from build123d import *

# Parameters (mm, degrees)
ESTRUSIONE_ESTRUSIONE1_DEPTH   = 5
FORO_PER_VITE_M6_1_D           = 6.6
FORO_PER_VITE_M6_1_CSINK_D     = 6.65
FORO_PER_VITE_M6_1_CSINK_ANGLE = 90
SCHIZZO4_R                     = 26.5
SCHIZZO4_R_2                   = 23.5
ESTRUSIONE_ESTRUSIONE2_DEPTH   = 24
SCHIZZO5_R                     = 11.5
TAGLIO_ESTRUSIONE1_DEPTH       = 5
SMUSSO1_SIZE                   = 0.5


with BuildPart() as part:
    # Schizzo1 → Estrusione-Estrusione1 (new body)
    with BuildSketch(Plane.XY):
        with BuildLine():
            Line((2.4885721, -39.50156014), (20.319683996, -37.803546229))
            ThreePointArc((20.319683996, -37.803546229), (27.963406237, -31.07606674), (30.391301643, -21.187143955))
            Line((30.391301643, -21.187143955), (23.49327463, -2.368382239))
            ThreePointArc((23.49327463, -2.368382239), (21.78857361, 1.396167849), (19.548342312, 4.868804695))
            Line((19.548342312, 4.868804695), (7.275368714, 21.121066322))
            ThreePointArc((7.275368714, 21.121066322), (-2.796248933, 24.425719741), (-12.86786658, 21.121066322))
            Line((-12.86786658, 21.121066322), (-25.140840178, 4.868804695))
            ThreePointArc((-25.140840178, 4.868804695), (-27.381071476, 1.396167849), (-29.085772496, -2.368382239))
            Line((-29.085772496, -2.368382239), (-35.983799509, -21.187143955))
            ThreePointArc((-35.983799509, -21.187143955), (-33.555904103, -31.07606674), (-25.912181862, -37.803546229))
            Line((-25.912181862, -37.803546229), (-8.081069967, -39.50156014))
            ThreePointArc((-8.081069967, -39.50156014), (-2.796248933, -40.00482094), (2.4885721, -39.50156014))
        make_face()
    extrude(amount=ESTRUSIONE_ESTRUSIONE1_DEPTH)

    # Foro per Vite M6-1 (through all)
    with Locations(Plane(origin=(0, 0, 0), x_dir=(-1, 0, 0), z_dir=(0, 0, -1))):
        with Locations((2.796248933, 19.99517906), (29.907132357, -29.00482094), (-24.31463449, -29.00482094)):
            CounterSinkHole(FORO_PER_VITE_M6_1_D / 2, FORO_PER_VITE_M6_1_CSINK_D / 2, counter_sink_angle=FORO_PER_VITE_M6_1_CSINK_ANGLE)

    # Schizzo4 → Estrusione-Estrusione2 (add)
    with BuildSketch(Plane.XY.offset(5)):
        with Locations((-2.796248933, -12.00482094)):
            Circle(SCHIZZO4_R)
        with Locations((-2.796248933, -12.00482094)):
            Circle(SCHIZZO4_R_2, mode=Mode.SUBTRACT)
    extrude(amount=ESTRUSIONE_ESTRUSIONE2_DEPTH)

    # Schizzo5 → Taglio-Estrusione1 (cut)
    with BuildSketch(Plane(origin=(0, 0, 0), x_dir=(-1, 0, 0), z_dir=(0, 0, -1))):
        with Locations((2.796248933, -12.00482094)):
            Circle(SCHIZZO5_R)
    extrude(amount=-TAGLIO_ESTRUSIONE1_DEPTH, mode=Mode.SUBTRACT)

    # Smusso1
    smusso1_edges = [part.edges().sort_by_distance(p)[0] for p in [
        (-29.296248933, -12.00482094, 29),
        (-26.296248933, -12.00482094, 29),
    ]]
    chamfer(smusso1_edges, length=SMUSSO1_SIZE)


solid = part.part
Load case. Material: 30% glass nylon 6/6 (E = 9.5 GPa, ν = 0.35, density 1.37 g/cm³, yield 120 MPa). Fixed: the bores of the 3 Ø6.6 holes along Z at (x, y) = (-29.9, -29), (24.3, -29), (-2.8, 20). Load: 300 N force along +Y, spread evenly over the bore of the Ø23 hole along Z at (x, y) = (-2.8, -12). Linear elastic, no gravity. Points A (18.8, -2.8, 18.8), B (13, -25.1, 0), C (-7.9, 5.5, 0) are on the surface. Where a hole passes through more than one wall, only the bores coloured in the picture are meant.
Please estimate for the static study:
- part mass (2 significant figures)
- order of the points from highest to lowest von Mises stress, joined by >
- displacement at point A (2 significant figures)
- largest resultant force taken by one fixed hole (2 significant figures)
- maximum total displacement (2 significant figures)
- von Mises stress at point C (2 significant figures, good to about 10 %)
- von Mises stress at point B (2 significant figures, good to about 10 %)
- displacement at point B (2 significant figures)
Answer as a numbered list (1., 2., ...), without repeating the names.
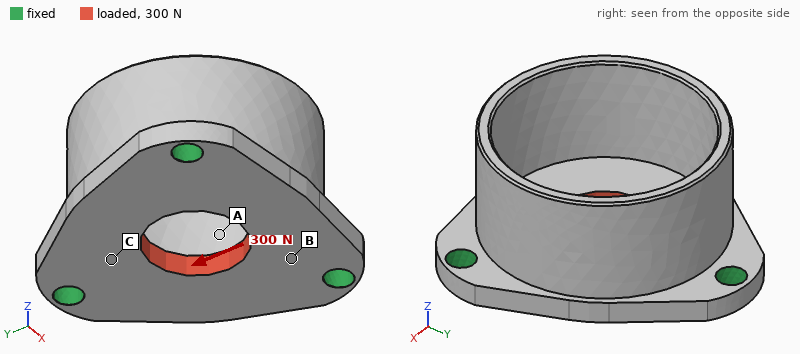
1. 33 g
2. C > B > A
3. 2.3 µm
4. 100 N
5. 6.7 µm
6. 1.3 MPa
7. 0.89 MPa
8. 3.1 µm
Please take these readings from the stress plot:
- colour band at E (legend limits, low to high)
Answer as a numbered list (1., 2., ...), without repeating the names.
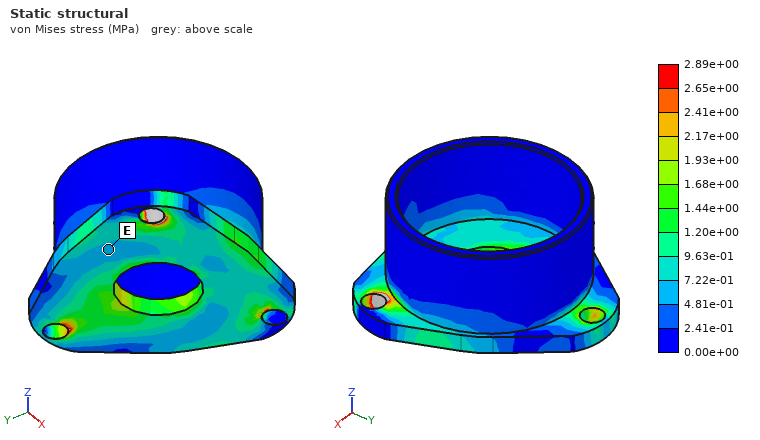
1. 4.81e-01 to 7.22e-01 MPa
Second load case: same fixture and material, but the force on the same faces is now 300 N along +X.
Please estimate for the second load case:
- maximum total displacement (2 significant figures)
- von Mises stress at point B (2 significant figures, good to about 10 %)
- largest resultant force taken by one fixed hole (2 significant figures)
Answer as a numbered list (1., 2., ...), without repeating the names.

1. 6.3 µm
2. 1.1 MPa
3. 100 N
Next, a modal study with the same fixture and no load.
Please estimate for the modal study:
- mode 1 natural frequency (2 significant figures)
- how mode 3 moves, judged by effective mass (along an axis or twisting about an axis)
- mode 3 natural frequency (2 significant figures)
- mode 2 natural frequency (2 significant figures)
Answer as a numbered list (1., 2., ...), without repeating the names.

1. 3000 Hz
2. along Z
3. 4900 Hz
4. 3000 Hz
